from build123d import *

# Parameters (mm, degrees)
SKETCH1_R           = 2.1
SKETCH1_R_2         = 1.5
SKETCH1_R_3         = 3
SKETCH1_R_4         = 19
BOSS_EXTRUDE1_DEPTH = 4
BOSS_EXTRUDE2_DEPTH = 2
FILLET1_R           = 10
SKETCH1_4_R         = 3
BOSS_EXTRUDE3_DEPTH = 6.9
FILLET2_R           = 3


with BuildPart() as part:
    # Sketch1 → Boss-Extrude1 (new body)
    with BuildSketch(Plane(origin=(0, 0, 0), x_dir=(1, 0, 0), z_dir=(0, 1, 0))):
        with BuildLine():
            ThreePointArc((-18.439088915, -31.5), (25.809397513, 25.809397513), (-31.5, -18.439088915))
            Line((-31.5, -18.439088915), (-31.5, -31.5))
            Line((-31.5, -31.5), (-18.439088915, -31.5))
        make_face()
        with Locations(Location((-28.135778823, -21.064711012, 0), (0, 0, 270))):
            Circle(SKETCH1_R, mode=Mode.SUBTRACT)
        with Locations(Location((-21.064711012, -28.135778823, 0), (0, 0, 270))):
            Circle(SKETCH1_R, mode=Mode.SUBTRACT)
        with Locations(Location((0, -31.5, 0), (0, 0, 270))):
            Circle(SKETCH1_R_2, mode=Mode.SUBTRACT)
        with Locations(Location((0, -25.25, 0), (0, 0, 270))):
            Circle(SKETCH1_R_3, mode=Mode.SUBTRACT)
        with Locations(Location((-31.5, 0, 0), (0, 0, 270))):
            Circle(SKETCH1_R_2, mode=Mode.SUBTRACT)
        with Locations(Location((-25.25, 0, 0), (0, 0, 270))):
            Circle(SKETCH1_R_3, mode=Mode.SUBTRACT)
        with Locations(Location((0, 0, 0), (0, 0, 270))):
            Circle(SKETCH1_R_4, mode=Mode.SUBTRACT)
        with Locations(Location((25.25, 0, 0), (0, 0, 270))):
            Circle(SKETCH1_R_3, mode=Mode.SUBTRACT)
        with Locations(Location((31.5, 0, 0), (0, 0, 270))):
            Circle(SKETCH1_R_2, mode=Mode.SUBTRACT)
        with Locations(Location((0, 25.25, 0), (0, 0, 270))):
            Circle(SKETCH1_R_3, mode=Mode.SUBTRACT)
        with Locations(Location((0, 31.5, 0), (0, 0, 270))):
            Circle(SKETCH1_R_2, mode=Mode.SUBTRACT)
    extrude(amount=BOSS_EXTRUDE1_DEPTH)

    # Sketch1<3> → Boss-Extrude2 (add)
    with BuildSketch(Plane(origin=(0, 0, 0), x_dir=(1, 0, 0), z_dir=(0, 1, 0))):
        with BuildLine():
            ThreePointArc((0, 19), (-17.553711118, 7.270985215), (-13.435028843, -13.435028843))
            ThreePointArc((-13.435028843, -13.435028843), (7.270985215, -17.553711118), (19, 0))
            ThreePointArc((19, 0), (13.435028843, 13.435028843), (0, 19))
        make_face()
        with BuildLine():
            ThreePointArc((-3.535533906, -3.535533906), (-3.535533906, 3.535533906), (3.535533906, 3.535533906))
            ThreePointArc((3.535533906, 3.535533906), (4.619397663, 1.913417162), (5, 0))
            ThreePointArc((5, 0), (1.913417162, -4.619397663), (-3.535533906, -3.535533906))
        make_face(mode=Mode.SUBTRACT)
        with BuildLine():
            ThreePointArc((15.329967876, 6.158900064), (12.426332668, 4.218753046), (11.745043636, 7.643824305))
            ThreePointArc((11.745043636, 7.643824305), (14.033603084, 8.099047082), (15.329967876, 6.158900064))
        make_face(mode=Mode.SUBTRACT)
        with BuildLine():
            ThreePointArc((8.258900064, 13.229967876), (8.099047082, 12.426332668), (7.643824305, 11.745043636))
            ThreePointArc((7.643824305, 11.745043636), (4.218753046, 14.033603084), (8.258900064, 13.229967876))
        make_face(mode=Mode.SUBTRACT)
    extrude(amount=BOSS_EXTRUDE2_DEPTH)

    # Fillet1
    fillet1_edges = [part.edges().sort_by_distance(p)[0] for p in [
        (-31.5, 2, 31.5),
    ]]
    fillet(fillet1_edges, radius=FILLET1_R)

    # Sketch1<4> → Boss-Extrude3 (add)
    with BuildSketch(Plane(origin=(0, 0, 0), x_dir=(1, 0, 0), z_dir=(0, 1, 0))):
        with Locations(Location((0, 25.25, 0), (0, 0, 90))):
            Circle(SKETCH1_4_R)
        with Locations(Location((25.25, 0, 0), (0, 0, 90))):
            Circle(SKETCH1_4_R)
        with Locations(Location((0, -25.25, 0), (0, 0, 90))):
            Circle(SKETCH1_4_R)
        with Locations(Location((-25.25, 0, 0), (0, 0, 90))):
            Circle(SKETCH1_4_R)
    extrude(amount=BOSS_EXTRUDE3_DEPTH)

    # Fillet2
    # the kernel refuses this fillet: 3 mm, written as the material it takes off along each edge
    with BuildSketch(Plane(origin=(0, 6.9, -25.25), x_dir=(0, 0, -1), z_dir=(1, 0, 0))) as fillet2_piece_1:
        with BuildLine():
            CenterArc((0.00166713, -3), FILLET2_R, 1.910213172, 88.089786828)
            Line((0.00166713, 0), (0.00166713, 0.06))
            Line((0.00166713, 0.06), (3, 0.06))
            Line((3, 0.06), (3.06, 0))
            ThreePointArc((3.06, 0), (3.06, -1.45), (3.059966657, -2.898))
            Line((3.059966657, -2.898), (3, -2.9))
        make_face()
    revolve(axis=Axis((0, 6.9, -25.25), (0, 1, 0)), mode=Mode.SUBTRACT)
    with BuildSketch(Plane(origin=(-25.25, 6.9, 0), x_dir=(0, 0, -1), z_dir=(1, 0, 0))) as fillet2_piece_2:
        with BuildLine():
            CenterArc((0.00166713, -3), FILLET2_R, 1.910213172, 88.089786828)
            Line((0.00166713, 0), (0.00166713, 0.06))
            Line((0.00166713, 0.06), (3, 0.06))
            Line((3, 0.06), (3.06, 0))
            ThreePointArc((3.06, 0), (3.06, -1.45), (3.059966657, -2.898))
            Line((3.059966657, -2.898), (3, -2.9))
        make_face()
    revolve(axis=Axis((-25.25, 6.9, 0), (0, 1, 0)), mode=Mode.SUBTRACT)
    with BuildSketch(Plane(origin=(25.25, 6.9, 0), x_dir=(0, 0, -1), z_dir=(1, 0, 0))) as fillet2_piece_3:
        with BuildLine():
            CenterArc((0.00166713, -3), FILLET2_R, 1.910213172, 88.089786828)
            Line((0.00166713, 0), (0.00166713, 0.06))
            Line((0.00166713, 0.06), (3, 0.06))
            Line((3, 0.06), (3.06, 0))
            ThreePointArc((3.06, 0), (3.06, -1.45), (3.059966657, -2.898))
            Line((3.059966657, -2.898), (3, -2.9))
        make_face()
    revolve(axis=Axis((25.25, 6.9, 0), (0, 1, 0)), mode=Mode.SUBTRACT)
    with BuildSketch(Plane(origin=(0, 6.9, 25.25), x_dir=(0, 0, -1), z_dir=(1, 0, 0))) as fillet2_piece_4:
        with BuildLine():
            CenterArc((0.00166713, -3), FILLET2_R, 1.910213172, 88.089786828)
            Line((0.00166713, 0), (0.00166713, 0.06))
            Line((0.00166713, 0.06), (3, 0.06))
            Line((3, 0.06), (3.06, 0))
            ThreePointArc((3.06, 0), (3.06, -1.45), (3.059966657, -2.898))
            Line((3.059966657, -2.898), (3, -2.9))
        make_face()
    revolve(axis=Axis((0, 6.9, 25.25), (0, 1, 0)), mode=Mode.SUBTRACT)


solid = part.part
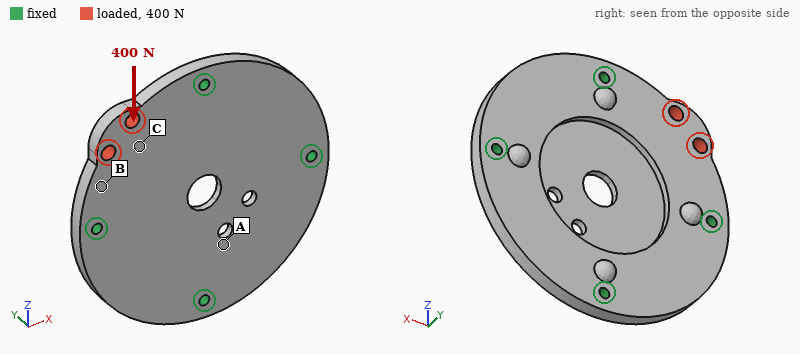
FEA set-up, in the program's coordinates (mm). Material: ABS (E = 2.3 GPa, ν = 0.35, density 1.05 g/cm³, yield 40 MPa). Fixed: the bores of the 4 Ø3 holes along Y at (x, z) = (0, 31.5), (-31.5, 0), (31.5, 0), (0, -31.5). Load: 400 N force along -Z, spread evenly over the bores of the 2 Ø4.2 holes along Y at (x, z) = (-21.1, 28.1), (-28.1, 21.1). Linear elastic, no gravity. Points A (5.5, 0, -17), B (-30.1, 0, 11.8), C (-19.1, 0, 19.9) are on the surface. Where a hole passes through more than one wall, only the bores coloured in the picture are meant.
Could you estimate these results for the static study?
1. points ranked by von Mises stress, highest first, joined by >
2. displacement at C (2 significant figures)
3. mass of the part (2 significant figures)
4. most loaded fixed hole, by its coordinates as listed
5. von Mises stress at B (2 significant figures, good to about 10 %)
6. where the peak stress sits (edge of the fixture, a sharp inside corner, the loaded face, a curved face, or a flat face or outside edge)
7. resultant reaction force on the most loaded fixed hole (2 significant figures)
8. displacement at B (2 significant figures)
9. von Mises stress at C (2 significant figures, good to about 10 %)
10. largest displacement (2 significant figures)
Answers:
B > C > A
47 µm
15 g
(-31.5, 0)
5.7 MPa
the loaded face
250 N
31 µm
3.0 MPa
95 µm
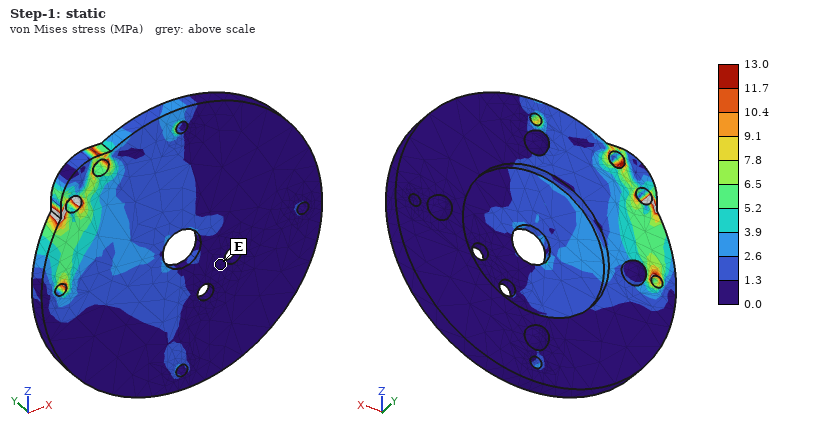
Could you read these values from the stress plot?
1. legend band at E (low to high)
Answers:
0.0 to 1.3 MPa
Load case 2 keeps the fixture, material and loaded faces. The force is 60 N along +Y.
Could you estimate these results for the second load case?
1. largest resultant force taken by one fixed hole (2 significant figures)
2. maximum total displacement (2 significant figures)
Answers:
35 N
0.50 mm
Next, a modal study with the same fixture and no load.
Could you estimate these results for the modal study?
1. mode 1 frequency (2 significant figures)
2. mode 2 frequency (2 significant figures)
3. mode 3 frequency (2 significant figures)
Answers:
2100 Hz
2200 Hz
2300 Hz
